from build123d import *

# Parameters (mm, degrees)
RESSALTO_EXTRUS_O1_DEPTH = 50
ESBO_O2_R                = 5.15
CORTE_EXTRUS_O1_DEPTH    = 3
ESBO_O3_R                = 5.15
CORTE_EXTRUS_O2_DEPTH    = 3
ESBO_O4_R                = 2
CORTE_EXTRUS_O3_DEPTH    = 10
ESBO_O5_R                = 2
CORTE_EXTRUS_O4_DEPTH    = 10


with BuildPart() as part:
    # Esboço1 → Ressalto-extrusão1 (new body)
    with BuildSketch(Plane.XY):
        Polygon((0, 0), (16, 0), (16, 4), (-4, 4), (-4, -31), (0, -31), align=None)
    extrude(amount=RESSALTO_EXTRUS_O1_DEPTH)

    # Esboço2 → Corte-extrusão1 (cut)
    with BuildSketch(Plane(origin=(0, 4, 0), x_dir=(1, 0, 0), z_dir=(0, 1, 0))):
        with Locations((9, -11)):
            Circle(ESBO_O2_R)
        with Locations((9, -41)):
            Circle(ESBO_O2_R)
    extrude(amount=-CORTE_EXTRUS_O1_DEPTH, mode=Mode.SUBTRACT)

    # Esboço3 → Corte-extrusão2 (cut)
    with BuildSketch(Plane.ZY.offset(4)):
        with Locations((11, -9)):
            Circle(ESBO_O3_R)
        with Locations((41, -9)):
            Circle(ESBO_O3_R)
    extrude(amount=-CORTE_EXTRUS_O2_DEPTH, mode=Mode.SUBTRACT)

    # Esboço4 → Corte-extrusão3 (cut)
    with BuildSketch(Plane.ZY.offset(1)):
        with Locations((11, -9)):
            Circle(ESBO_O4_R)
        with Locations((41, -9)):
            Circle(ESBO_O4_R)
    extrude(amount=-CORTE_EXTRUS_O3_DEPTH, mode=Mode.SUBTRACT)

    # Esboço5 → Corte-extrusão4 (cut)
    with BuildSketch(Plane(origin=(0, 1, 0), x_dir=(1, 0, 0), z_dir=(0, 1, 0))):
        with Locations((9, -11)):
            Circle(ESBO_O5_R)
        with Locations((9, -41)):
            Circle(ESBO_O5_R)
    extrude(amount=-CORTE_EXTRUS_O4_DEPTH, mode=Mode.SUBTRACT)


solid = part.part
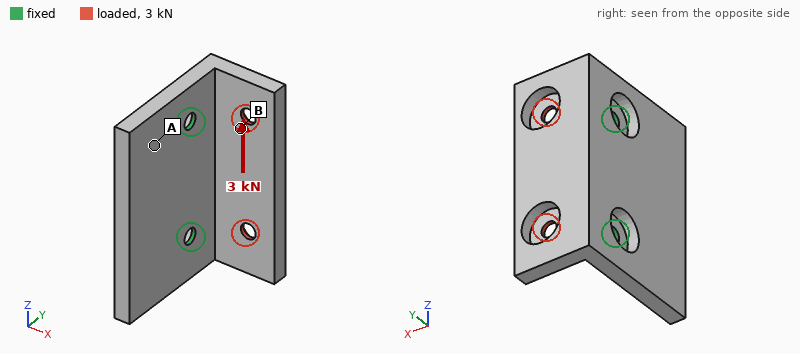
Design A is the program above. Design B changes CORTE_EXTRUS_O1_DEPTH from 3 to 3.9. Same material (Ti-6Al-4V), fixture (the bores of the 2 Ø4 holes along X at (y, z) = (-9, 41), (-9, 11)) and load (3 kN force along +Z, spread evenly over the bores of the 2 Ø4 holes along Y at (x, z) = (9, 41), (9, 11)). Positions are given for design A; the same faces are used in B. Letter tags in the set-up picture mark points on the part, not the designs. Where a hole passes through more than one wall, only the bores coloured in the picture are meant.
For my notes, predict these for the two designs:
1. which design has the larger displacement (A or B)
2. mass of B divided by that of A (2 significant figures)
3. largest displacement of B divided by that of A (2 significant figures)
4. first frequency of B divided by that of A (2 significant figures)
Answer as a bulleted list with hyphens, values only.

- B
- 0.99
- 1.1
- 1.0
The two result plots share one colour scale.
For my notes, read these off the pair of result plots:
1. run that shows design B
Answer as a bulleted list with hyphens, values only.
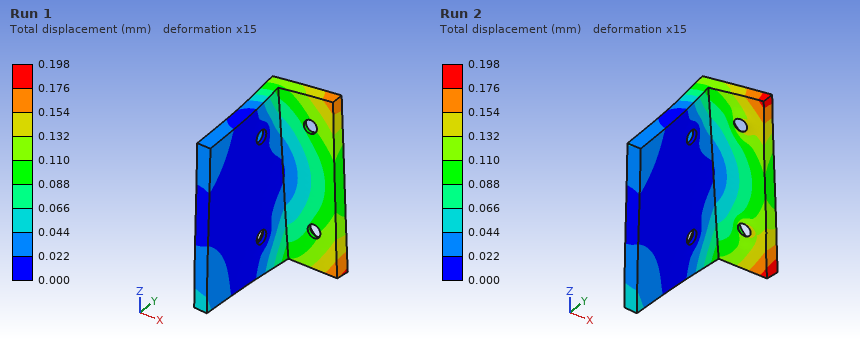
- Run 2
